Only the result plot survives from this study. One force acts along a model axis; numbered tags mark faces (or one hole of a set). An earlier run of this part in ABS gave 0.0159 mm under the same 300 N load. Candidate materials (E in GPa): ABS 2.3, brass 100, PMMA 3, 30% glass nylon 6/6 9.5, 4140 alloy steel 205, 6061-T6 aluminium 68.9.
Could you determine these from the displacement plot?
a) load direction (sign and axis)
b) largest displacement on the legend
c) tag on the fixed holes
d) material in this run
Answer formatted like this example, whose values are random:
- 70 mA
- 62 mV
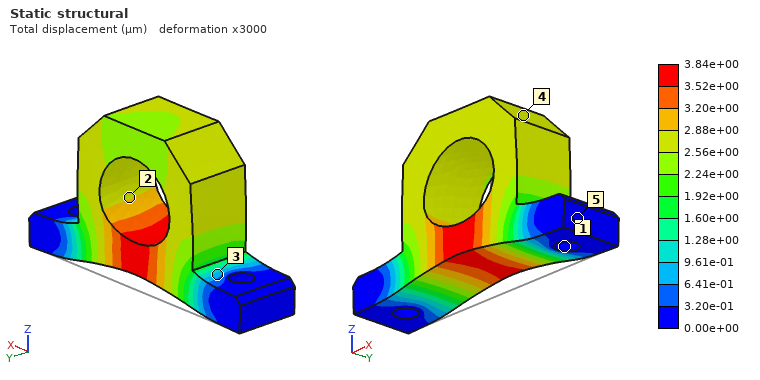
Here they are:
- +Z
- 3.84e+00 µm
- 1
- 30% glass nylon 6/6
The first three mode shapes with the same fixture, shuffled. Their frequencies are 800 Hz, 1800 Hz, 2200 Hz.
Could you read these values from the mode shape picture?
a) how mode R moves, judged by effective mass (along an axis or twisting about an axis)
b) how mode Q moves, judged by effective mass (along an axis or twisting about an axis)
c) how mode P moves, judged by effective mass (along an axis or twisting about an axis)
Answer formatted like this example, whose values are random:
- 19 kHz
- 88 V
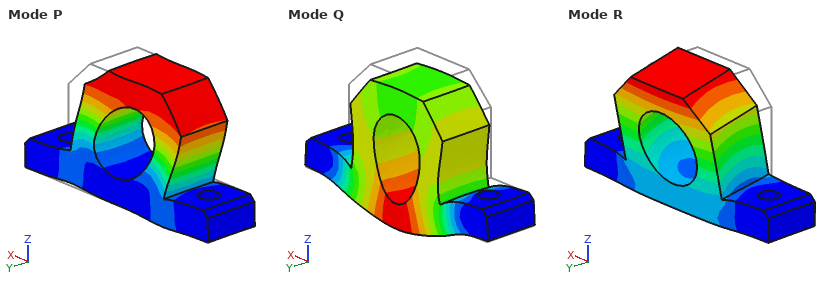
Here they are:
- along Y
- along Z
- along X
